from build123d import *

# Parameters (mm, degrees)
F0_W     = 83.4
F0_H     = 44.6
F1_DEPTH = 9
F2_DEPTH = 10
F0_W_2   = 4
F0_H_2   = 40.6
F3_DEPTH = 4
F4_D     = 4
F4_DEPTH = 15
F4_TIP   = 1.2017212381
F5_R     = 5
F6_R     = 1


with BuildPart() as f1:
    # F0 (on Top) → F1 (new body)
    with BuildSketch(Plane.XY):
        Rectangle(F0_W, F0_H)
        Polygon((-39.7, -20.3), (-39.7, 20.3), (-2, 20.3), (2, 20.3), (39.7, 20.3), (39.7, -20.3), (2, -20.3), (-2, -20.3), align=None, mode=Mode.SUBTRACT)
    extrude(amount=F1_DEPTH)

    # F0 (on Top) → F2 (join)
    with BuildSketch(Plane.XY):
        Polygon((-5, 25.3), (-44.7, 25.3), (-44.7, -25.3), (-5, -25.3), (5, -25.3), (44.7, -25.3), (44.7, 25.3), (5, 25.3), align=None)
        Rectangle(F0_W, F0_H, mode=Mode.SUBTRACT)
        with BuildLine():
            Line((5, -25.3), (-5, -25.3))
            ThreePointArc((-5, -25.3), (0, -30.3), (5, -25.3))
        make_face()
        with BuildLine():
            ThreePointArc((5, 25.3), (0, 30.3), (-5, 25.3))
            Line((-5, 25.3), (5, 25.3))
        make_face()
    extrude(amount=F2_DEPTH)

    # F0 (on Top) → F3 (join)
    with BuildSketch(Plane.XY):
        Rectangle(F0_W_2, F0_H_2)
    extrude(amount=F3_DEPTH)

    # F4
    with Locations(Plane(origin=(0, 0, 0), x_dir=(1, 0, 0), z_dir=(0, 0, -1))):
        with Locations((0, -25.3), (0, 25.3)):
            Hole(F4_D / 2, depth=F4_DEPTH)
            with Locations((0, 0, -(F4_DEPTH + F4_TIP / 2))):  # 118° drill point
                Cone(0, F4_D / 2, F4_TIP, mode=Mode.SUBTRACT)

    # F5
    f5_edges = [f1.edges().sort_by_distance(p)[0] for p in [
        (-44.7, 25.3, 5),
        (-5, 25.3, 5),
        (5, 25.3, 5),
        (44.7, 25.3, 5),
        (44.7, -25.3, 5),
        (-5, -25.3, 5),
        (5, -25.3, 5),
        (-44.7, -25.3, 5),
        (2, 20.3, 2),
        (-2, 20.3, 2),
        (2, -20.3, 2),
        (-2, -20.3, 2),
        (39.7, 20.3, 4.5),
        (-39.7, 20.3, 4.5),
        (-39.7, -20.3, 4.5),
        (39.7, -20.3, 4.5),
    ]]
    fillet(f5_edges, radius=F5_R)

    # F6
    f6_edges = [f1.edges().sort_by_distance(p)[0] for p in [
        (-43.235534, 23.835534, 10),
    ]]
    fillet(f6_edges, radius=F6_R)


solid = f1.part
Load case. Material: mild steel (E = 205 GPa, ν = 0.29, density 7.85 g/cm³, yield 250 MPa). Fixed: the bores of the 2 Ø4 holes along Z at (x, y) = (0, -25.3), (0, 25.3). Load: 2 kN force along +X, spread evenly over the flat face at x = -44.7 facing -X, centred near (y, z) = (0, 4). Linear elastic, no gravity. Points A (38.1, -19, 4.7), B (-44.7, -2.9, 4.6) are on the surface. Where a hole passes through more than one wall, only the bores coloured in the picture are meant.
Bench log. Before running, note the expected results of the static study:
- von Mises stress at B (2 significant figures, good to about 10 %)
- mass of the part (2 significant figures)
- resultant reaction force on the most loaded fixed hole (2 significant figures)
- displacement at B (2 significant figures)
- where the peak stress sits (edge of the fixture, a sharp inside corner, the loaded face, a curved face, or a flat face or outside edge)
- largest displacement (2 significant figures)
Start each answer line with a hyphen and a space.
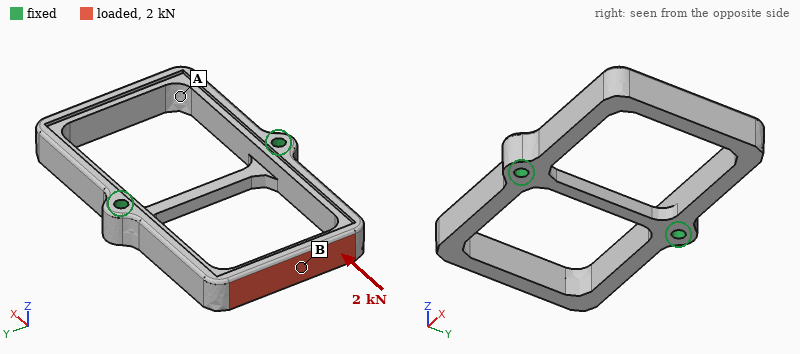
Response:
- 140 MPa
- 110 g
- 1.0 kN
- 50 µm
- a curved face
- 52 µm
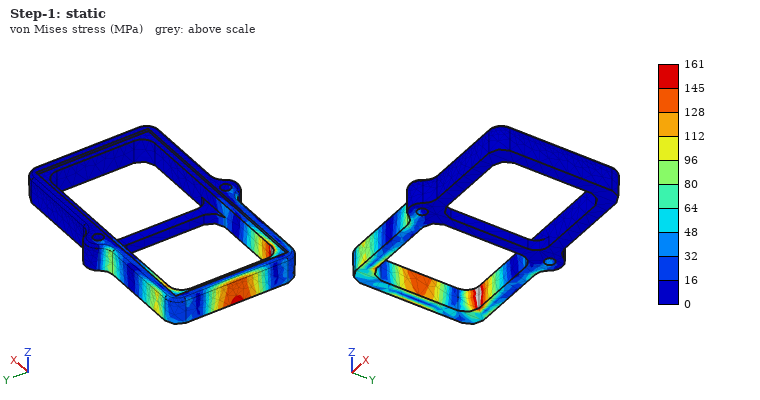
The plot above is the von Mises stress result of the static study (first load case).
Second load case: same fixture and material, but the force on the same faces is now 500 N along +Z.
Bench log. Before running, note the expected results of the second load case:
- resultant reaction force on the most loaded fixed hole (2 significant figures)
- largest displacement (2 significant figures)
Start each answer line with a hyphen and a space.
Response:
- 250 N
- 97 µm
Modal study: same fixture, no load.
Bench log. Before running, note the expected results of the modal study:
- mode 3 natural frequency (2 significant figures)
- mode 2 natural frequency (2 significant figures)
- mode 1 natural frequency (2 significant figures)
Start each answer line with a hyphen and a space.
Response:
- 2600 Hz
- 2600 Hz
- 2500 Hz
